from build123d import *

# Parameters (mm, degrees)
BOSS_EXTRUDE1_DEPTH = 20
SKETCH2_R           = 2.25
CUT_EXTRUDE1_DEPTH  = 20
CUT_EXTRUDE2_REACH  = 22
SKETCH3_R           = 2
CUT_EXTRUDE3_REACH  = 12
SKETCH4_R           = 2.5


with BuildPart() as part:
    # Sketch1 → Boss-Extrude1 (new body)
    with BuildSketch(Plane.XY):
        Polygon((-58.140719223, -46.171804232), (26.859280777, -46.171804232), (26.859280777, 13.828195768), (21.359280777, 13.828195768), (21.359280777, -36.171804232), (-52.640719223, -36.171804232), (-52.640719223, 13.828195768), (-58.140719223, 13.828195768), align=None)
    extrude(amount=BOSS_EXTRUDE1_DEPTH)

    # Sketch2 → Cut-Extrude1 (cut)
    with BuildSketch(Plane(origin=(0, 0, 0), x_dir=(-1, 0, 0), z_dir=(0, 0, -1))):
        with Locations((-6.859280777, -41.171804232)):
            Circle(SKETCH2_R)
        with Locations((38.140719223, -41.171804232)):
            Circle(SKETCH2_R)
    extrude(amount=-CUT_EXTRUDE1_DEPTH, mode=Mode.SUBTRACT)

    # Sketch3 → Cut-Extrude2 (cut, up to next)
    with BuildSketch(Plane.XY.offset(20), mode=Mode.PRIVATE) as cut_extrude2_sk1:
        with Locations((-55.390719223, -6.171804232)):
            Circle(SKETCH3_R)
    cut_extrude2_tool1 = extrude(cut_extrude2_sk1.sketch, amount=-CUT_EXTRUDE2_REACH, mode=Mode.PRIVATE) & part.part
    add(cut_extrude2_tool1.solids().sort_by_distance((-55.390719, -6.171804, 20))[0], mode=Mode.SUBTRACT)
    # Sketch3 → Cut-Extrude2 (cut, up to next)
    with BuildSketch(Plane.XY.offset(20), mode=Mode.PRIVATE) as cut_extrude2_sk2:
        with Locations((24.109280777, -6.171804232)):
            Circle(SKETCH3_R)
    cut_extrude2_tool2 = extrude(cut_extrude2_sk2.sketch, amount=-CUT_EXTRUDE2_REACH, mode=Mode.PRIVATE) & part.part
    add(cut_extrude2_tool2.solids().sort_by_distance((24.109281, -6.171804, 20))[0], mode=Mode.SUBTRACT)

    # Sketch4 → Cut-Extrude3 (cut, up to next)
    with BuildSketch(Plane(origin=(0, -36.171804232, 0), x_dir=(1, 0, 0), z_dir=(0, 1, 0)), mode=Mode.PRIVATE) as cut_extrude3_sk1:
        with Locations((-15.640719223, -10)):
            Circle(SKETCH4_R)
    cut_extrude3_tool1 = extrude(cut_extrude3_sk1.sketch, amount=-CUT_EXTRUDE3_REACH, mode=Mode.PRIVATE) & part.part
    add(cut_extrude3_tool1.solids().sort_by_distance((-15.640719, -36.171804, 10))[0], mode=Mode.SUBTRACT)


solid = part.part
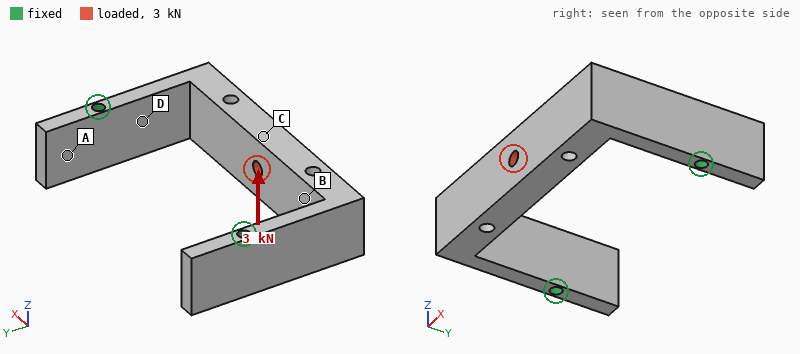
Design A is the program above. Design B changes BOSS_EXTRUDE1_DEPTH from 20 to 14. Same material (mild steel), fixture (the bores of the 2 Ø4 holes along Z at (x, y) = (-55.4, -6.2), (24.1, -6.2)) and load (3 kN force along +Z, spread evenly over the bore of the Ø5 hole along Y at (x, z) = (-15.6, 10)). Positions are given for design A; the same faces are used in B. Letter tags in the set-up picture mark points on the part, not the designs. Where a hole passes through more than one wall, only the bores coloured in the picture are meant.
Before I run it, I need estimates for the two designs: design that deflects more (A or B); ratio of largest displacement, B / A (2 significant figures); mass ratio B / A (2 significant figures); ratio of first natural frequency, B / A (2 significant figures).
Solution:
B
2.7
0.70
1.00
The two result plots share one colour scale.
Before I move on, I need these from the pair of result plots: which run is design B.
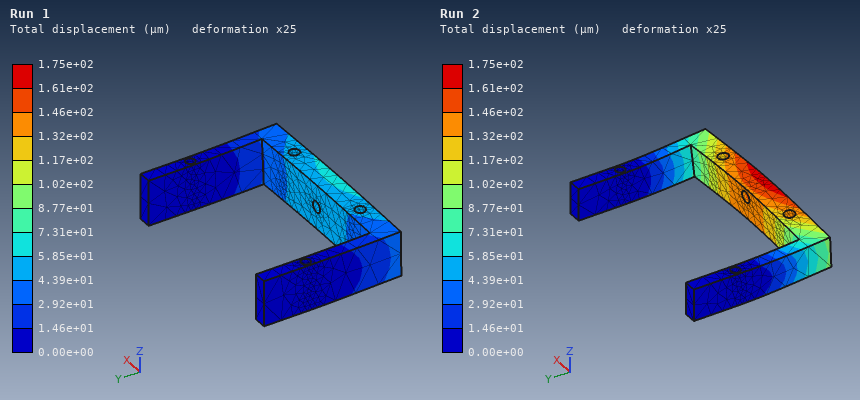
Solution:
Run 2
